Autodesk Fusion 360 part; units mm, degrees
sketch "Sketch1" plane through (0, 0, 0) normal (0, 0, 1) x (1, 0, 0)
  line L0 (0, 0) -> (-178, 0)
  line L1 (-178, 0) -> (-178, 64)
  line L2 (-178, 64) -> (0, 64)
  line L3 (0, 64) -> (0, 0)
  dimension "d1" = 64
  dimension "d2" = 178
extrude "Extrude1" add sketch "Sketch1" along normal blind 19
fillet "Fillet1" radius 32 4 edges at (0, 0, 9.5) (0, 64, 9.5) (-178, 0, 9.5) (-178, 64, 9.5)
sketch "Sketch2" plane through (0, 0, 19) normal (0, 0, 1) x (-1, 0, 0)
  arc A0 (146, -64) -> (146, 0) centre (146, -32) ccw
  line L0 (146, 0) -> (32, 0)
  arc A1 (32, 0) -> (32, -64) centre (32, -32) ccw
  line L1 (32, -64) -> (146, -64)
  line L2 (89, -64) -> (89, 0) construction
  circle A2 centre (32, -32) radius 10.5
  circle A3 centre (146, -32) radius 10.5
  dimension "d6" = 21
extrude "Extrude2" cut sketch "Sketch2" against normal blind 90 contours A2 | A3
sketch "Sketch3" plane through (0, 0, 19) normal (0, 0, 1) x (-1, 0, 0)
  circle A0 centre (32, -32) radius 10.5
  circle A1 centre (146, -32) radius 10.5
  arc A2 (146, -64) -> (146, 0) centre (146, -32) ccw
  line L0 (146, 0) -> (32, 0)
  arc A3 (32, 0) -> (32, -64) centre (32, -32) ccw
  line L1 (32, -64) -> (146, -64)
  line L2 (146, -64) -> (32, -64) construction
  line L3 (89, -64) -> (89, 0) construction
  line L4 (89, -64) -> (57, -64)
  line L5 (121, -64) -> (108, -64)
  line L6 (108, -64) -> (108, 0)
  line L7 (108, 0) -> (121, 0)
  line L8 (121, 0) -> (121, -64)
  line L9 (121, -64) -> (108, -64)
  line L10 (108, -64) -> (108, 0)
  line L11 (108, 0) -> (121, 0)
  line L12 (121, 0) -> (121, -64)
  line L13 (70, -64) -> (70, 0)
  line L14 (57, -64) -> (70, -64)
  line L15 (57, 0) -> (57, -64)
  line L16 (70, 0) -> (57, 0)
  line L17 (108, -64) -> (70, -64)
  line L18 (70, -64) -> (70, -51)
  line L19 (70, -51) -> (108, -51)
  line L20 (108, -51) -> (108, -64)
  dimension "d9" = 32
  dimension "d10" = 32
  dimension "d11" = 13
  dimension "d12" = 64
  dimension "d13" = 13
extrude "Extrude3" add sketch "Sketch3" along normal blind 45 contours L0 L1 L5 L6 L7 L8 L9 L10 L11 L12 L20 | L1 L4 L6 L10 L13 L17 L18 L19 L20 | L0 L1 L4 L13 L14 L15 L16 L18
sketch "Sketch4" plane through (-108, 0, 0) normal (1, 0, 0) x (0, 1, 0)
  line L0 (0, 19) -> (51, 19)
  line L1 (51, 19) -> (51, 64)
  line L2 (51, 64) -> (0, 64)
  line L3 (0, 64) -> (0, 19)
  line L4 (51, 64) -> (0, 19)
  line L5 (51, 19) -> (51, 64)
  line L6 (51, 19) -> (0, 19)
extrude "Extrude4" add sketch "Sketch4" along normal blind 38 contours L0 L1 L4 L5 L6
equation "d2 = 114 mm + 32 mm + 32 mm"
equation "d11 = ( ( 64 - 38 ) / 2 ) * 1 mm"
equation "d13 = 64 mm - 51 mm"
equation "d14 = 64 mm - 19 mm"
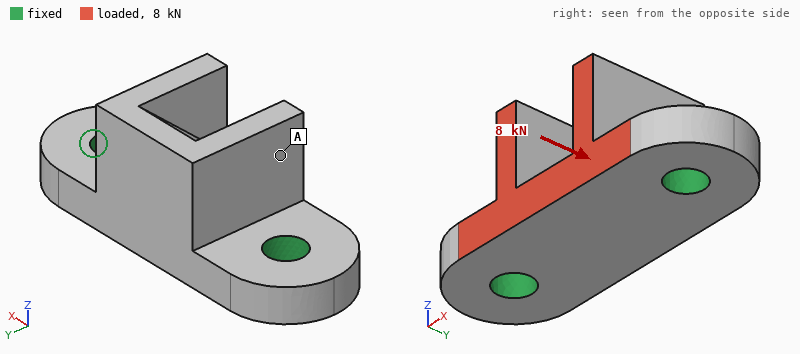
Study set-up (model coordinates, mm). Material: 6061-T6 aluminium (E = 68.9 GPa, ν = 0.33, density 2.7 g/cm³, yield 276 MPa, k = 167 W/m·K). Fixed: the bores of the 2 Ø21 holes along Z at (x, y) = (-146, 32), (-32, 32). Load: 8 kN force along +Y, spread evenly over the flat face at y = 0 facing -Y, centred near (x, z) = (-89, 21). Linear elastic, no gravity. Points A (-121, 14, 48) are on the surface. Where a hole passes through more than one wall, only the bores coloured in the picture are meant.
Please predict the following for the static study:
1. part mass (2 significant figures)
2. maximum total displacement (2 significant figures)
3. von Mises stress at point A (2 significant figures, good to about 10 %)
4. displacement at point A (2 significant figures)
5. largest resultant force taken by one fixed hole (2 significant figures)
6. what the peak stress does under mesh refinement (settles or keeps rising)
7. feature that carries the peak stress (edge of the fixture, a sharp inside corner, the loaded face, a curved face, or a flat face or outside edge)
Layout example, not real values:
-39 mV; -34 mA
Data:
880 g; 25 µm; 2.6 MPa; 18 µm; 4.0 kN; keeps rising; edge of the fixture
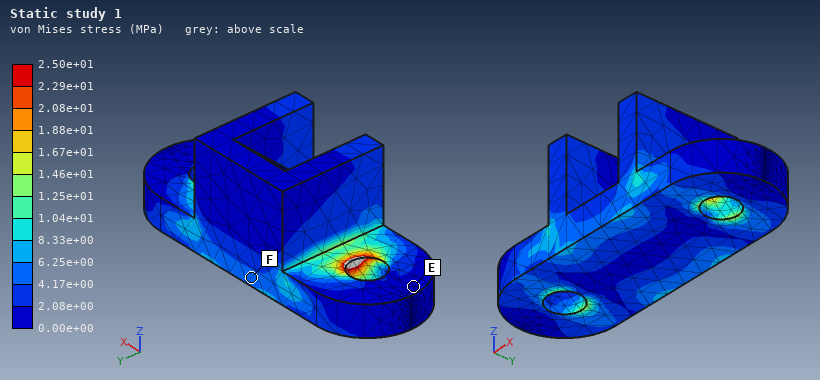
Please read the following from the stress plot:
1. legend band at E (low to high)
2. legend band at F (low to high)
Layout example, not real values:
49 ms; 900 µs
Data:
0.00e+00 to 2.08e+00 MPa; 4.17e+00 to 6.25e+00 MPa
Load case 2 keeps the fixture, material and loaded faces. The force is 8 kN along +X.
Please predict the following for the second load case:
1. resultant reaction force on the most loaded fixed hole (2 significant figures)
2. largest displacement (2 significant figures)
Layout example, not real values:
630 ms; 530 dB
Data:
4.6 kN; 31 µm
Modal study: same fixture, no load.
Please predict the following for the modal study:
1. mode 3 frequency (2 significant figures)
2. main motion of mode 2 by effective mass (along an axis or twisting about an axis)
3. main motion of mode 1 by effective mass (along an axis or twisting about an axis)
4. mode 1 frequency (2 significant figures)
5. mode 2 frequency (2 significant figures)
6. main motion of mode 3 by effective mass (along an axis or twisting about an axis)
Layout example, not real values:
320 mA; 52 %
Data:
7000 Hz; along Z; along Y; 3400 Hz; 6100 Hz; along X
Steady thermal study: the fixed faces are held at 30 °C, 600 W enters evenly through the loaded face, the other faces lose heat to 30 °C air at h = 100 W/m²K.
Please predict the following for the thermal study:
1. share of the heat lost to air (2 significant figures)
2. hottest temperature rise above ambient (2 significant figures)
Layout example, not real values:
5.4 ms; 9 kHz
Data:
15 %; 63 K
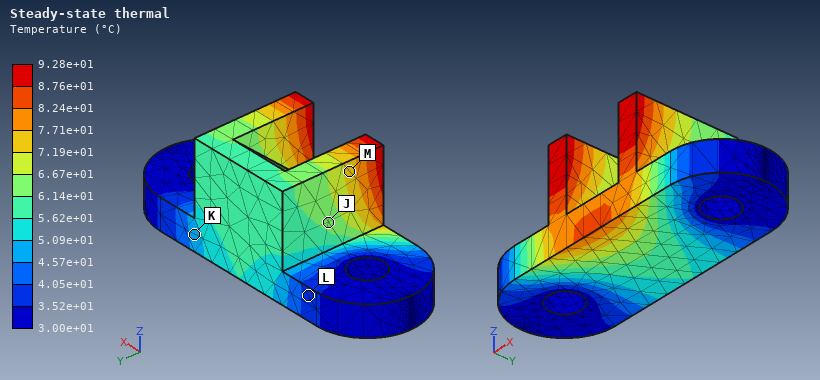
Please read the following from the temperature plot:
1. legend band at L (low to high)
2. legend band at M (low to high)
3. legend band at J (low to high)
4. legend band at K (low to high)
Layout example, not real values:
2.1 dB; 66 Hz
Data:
3.52e+01 to 4.05e+01 °C; 7.19e+01 to 7.71e+01 °C; 6.14e+01 to 6.67e+01 °C; 4.57e+01 to 5.09e+01 °C
